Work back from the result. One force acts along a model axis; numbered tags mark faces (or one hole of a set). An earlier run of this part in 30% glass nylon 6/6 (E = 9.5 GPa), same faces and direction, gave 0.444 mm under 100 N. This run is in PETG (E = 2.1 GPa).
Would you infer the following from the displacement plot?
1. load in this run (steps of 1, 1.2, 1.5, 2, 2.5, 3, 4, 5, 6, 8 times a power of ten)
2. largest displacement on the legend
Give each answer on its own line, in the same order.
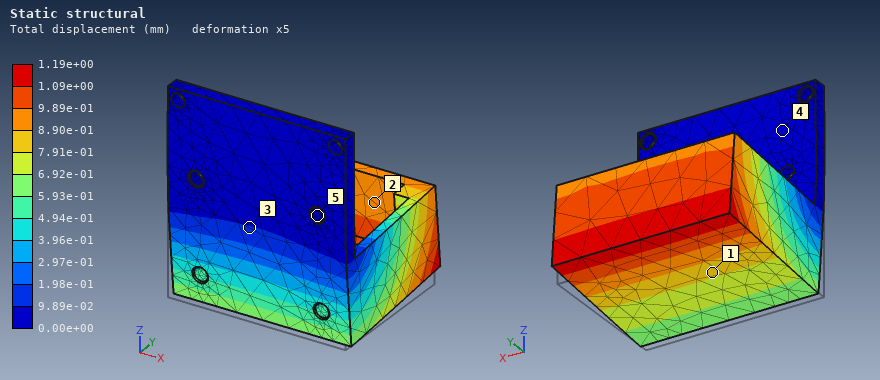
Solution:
60 N
1.19e+00 mm
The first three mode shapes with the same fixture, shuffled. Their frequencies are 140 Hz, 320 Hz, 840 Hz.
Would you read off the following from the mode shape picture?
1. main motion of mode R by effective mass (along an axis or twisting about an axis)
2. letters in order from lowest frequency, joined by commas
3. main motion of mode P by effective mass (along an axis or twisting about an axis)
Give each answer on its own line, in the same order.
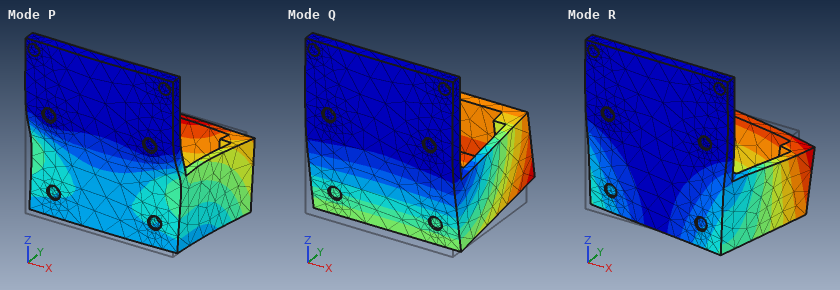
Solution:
along X
Q, R, P
along Y
